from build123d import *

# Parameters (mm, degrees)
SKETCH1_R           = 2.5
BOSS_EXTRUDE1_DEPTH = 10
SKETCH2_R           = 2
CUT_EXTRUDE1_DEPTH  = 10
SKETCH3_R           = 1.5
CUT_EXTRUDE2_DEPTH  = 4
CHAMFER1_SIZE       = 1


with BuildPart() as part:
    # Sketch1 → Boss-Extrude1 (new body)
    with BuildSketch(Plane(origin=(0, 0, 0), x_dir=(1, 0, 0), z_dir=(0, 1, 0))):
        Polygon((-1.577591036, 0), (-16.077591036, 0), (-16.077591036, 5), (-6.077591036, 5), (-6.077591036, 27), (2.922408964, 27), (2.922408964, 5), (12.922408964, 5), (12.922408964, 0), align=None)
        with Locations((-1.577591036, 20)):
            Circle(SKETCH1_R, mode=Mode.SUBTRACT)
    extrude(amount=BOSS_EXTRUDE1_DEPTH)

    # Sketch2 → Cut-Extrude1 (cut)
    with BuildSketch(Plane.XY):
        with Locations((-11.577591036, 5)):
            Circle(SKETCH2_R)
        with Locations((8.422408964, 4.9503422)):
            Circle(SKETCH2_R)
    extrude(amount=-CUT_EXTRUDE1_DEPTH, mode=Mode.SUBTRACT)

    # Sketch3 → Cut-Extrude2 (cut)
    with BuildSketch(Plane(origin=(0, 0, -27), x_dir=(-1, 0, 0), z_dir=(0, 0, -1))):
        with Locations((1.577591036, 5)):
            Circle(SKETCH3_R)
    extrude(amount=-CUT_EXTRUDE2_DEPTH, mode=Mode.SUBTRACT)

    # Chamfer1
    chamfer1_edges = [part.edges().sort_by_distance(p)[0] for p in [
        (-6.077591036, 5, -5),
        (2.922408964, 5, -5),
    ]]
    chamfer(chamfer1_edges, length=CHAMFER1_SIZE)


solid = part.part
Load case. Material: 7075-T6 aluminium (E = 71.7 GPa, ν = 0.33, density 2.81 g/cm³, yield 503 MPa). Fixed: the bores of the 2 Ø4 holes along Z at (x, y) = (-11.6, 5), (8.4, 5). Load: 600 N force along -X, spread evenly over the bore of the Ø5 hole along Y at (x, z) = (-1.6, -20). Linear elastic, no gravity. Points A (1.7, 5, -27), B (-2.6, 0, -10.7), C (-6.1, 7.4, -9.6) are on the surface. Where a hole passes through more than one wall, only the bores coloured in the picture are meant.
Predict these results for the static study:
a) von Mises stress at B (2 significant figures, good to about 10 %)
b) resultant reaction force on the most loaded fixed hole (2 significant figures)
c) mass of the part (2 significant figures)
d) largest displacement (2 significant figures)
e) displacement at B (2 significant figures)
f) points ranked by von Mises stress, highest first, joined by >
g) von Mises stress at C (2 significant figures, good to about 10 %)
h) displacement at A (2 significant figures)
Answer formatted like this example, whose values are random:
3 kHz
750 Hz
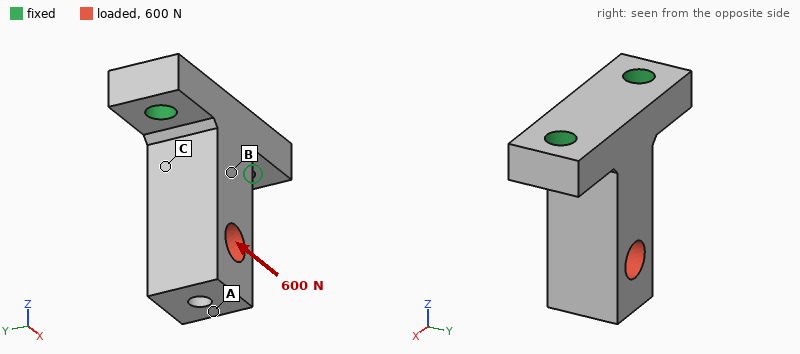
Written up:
21 MPa
760 N
8.7 g
53 µm
9.5 µm
C > B > A
46 MPa
53 µm
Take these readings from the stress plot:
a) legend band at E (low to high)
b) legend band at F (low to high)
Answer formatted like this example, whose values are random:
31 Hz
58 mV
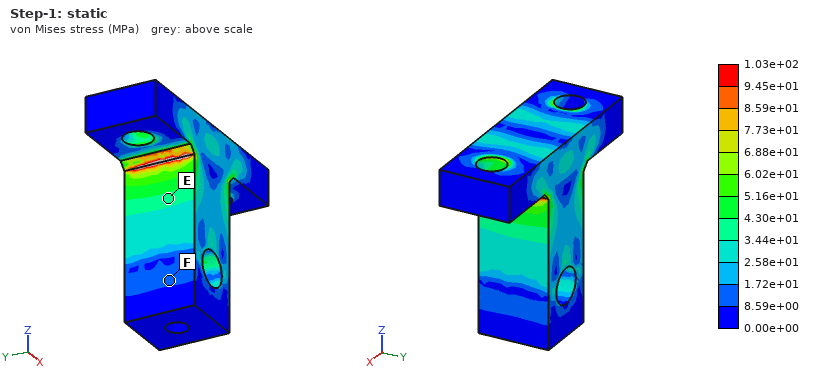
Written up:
3.44e+01 to 4.30e+01 MPa
8.59e+00 to 1.72e+01 MPa
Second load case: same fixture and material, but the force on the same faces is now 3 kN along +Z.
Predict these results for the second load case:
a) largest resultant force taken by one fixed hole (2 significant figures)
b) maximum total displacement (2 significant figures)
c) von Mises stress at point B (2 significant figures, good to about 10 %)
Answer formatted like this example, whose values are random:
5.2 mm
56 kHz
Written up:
1.6 kN
24 µm
30 MPa
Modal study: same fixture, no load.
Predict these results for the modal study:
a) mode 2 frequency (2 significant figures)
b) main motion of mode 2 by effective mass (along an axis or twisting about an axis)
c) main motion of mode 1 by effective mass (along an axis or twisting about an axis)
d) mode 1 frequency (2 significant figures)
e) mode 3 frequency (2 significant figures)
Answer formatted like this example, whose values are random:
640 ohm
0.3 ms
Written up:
11 kHz
along X
along Y
7600 Hz
30 kHz
